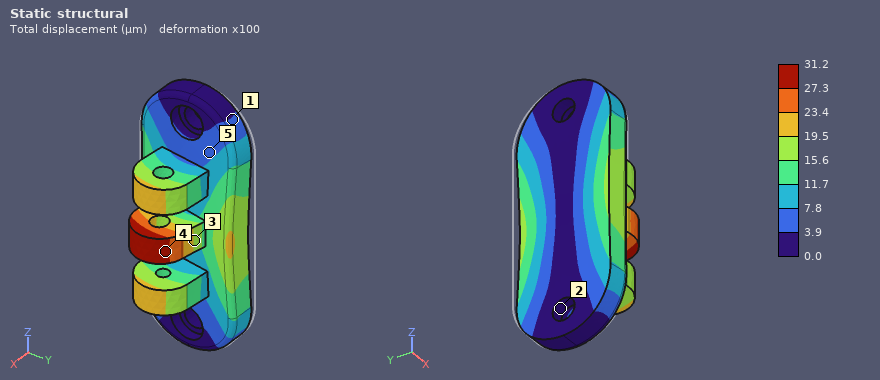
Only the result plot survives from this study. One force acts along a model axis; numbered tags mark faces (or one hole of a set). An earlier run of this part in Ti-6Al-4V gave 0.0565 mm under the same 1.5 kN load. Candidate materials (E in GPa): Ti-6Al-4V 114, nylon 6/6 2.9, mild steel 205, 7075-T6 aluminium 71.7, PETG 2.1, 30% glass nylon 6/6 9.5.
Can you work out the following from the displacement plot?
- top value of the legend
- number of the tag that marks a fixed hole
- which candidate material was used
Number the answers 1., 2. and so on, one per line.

1. 31.2 µm
2. 2
3. mild steel
